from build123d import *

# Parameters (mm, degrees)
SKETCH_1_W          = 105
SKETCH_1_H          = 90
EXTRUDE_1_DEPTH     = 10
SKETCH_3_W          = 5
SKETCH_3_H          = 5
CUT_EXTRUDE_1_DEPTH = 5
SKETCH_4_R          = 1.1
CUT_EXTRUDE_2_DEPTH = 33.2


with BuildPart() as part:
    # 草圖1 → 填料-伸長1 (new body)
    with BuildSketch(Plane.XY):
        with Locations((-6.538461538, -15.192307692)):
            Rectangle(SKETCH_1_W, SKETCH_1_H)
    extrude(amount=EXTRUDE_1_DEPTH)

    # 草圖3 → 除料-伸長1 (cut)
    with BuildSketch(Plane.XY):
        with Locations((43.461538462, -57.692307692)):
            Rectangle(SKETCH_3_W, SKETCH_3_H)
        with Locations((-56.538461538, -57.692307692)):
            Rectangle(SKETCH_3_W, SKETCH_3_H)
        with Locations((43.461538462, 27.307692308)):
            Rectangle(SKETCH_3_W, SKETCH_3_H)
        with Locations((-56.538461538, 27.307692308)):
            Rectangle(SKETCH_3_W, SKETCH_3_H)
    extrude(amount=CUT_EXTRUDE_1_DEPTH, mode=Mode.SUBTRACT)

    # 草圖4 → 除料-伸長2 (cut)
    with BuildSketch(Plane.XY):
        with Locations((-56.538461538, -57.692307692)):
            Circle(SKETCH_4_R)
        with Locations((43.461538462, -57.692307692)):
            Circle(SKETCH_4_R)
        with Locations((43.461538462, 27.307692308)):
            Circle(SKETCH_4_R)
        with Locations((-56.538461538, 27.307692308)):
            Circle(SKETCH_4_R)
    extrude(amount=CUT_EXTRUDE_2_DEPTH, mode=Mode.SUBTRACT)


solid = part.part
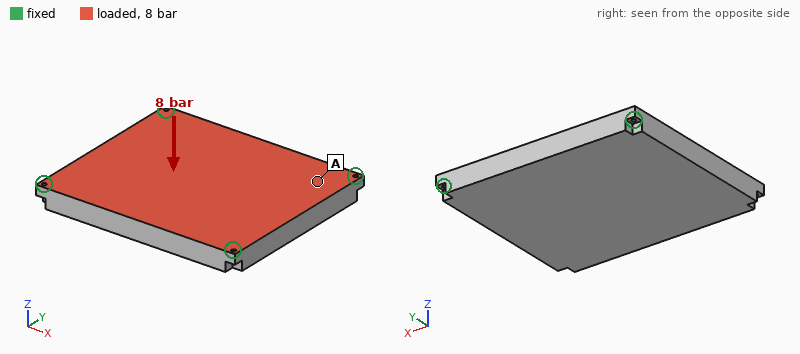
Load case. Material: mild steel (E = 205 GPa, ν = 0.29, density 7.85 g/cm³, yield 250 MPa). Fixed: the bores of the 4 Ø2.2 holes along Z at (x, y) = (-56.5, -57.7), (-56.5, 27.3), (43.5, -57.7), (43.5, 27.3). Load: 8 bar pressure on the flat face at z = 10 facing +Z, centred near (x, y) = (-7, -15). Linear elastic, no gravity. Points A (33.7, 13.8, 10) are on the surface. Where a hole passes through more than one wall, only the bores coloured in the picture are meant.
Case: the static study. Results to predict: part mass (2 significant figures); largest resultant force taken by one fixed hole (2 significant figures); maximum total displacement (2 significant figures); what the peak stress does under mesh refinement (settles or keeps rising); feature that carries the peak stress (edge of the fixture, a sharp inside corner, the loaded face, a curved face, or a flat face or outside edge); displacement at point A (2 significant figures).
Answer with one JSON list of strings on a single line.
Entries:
["740 g", "3.1 kN", "57 µm", "keeps rising", "edge of the fixture", "24 µm"]
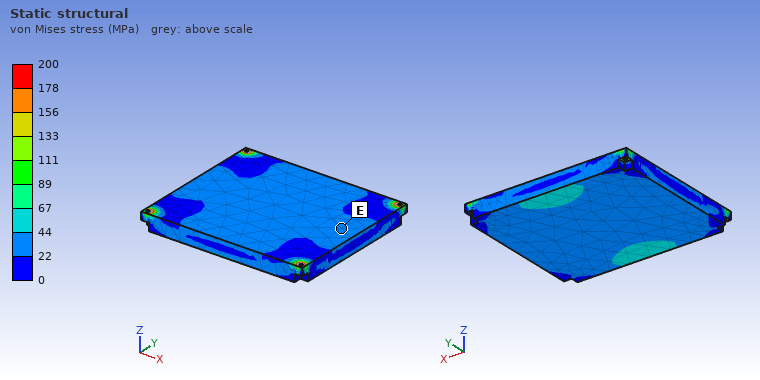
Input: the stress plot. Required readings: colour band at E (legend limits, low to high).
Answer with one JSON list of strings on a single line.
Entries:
["22 to 44 MPa"]
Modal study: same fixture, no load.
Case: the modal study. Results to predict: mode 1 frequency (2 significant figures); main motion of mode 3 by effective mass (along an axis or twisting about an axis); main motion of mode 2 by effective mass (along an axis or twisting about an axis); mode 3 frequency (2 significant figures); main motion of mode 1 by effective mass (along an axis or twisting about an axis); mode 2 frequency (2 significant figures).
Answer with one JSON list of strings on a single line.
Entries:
["2400 Hz", "twisting about Y", "twisting about X", "5000 Hz", "along Z", "4500 Hz"]
